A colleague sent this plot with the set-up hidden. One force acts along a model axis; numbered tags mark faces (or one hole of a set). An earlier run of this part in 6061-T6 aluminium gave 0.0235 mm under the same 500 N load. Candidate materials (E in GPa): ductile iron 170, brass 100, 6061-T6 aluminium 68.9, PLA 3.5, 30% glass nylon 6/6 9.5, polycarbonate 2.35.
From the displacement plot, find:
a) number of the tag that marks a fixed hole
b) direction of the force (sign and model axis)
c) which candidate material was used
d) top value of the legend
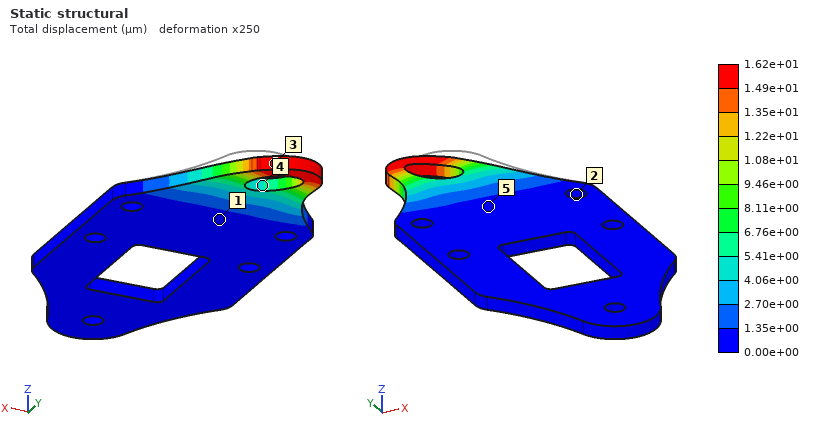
2
-X
brass
1.62e+01 µm
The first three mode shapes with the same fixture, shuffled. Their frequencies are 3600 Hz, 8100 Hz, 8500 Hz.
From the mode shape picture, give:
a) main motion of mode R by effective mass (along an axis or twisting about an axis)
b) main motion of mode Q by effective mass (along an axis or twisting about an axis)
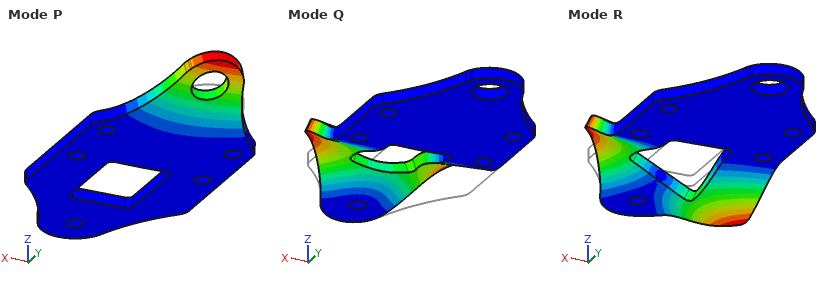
twisting about Y
along Z
